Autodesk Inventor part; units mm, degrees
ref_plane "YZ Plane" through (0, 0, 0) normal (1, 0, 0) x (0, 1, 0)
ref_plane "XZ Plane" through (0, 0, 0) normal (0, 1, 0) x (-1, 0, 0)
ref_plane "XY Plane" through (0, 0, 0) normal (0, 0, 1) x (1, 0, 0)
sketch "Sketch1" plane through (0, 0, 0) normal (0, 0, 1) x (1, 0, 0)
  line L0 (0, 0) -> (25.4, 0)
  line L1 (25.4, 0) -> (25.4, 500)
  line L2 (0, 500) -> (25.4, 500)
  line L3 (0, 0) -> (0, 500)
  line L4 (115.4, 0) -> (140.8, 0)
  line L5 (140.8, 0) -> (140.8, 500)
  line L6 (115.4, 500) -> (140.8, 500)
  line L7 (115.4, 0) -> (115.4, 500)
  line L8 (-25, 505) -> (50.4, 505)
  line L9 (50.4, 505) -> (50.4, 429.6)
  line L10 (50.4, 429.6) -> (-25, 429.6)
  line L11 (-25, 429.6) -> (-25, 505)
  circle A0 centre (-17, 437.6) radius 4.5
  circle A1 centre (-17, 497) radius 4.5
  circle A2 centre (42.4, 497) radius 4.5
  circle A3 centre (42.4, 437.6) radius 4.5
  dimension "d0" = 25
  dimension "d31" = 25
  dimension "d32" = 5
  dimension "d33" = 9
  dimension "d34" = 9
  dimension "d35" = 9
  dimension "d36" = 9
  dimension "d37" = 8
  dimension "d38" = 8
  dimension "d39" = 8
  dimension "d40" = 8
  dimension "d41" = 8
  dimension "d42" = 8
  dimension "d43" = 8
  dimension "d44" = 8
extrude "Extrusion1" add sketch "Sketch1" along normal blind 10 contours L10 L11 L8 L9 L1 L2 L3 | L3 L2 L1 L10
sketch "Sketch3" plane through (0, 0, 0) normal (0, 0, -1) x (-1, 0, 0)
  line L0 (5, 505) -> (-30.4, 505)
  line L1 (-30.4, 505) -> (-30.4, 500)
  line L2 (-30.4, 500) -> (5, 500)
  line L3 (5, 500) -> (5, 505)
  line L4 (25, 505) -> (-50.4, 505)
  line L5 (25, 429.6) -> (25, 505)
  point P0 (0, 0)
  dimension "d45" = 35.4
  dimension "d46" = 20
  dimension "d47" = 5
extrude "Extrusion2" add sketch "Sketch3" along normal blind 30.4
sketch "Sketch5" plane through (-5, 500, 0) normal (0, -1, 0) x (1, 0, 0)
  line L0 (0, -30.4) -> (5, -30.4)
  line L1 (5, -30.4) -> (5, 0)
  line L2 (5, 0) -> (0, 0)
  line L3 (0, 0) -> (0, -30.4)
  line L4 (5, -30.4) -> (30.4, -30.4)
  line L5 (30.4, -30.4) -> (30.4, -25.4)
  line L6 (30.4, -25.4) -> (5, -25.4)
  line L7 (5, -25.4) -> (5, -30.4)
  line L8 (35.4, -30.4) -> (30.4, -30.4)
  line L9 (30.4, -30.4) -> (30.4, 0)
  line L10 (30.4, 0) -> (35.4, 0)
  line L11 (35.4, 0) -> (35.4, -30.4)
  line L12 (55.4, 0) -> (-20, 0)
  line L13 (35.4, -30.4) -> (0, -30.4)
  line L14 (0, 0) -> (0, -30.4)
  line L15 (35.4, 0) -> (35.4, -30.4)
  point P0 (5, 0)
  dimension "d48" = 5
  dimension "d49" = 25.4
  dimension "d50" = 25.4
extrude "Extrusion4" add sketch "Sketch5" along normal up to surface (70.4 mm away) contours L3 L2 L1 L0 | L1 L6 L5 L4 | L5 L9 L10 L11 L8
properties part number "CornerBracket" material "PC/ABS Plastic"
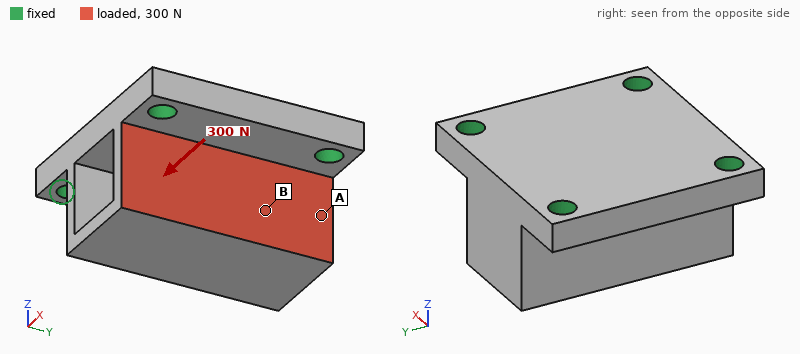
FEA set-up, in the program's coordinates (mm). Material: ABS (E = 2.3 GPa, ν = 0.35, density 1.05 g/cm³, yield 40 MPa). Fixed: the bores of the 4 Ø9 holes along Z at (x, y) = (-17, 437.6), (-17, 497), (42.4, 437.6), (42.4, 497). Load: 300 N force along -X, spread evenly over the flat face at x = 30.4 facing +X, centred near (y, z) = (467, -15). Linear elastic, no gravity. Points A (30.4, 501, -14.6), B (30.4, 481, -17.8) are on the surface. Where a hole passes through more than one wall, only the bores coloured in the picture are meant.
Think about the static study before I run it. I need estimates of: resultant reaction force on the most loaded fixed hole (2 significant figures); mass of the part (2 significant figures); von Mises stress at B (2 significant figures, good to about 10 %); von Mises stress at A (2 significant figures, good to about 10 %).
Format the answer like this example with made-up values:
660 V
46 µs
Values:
130 N
95 g
1.3 MPa
0.51 MPa
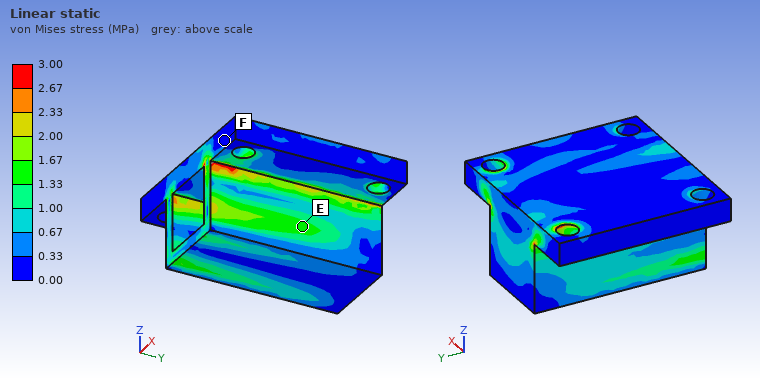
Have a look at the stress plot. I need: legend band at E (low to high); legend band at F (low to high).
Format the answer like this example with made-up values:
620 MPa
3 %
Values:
1.33 to 1.67 MPa
0.00 to 0.33 MPa
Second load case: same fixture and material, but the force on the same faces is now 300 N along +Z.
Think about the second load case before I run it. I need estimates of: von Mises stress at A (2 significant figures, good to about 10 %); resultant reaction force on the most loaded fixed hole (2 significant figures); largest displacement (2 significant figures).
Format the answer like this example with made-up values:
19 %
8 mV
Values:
0.59 MPa
140 N
36 µm
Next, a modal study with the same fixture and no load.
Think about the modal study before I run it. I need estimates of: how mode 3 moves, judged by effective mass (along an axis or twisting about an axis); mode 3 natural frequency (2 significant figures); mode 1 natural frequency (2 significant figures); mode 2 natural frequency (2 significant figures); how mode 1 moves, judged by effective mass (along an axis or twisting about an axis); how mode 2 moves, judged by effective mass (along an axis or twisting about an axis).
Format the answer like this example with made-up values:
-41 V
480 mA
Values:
along Z
2700 Hz
1500 Hz
2600 Hz
along X
along Y
